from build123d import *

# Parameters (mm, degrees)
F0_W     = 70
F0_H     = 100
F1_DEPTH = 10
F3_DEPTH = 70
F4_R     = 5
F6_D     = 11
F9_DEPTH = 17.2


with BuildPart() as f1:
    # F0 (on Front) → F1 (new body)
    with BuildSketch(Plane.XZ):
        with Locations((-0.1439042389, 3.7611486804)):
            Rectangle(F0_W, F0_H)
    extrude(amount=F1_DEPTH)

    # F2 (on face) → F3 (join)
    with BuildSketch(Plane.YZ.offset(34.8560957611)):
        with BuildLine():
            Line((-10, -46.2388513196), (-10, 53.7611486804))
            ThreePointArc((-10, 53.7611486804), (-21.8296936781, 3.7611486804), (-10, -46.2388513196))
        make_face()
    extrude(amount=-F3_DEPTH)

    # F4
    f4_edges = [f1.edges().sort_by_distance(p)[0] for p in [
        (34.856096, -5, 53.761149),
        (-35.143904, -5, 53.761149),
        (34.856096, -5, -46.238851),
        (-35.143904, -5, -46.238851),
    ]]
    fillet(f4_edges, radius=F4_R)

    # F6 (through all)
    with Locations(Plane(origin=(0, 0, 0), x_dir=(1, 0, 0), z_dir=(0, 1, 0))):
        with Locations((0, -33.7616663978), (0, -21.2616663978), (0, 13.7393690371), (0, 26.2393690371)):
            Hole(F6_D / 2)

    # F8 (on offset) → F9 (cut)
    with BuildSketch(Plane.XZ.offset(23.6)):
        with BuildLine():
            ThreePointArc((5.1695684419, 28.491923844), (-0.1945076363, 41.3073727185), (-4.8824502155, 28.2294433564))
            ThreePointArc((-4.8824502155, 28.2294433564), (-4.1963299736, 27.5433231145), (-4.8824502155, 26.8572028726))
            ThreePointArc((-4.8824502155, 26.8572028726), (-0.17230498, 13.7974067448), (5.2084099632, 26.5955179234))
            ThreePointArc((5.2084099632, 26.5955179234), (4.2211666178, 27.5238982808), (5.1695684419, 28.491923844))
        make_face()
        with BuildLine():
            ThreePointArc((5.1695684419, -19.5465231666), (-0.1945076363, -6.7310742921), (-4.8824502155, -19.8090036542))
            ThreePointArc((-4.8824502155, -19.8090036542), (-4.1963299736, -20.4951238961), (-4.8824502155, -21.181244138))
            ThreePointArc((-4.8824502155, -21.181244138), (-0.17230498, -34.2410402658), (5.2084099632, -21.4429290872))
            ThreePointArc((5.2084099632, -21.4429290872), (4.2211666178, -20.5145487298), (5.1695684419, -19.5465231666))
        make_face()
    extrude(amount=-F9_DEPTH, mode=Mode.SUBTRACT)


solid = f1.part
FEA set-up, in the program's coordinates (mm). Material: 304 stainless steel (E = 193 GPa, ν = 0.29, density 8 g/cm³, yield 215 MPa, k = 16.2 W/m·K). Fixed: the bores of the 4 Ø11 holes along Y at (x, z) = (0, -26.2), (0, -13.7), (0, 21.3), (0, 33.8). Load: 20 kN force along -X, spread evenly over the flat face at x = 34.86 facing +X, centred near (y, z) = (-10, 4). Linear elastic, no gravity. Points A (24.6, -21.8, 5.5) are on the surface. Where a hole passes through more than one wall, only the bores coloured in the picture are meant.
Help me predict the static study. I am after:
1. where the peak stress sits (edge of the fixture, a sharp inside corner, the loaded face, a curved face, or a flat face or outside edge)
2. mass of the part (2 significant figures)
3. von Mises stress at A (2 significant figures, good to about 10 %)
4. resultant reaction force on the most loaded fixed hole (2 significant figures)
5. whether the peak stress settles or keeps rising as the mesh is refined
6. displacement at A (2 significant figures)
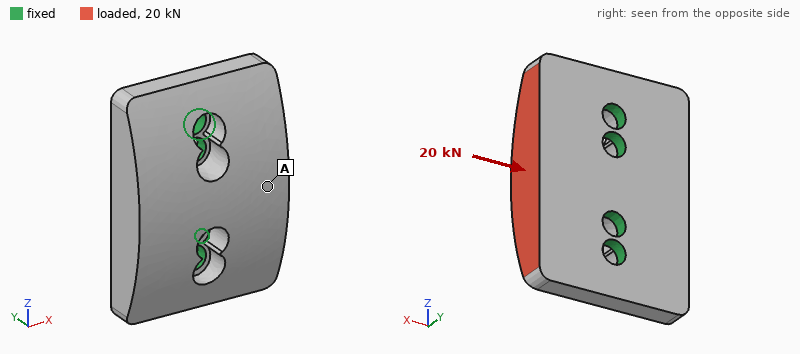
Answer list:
a sharp inside corner
920 g
17 MPa
5.4 kN
keeps rising
18 µm
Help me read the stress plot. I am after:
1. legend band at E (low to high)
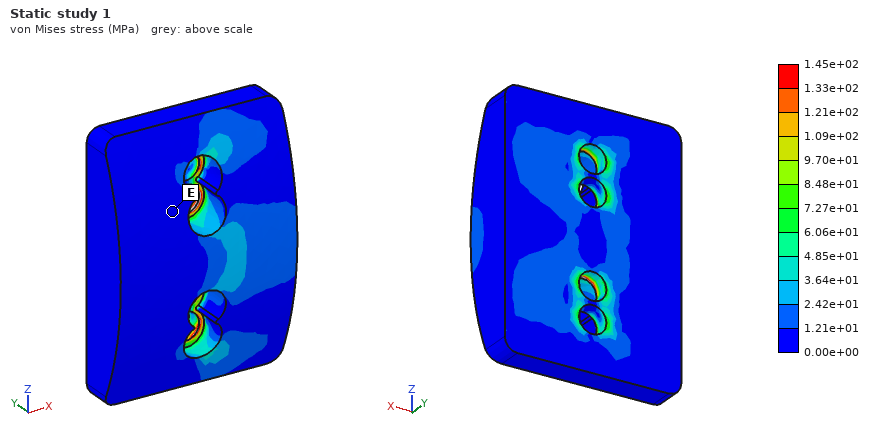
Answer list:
0.00e+00 to 1.21e+01 MPa
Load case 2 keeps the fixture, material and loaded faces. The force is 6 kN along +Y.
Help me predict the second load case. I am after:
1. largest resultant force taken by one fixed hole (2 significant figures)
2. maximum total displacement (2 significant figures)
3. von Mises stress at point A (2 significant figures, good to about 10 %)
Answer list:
2.1 kN
37 µm
18 MPa
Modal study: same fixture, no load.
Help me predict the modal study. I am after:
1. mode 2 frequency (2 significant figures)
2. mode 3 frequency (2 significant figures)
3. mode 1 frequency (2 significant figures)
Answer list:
8800 Hz
8800 Hz
4100 Hz
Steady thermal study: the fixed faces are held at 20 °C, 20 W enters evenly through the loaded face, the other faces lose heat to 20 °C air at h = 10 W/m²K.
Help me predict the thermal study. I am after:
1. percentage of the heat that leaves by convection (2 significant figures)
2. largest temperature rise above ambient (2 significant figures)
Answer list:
8.4 %
30 K
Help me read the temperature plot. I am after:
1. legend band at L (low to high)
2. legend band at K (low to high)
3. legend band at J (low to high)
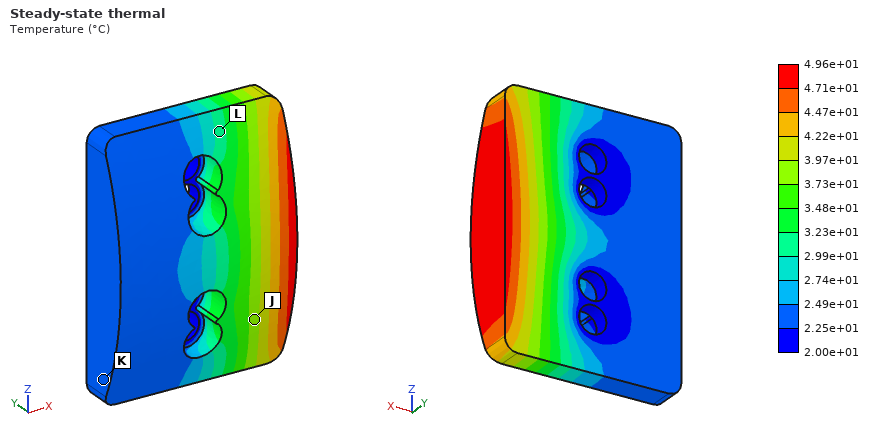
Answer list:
2.99e+01 to 3.23e+01 °C
2.25e+01 to 2.49e+01 °C
3.73e+01 to 3.97e+01 °C
